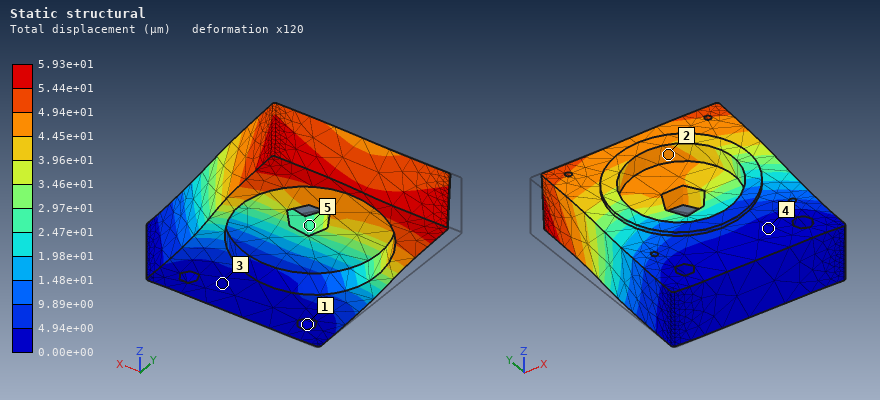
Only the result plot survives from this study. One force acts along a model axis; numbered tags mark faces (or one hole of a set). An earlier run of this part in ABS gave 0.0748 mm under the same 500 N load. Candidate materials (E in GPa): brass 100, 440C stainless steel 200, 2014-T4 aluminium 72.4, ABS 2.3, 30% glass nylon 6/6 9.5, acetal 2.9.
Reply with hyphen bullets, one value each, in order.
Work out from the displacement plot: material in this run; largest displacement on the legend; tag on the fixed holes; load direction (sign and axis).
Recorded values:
- acetal
- 5.93e+01 µm
- 1
- +X
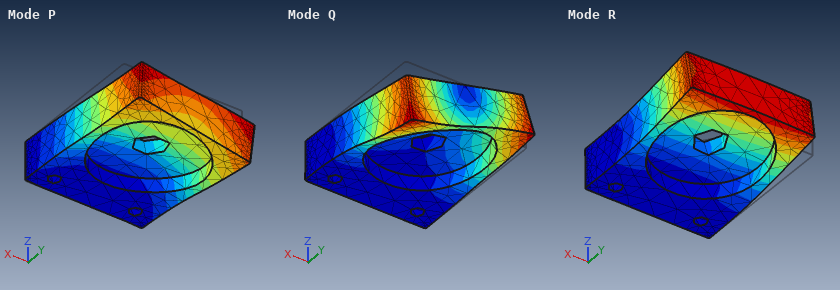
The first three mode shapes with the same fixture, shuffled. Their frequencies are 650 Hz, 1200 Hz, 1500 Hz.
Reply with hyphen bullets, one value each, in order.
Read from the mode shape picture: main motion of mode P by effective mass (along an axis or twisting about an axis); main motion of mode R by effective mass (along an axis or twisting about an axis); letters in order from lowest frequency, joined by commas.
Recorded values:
- along X
- along Z
- R, Q, P
